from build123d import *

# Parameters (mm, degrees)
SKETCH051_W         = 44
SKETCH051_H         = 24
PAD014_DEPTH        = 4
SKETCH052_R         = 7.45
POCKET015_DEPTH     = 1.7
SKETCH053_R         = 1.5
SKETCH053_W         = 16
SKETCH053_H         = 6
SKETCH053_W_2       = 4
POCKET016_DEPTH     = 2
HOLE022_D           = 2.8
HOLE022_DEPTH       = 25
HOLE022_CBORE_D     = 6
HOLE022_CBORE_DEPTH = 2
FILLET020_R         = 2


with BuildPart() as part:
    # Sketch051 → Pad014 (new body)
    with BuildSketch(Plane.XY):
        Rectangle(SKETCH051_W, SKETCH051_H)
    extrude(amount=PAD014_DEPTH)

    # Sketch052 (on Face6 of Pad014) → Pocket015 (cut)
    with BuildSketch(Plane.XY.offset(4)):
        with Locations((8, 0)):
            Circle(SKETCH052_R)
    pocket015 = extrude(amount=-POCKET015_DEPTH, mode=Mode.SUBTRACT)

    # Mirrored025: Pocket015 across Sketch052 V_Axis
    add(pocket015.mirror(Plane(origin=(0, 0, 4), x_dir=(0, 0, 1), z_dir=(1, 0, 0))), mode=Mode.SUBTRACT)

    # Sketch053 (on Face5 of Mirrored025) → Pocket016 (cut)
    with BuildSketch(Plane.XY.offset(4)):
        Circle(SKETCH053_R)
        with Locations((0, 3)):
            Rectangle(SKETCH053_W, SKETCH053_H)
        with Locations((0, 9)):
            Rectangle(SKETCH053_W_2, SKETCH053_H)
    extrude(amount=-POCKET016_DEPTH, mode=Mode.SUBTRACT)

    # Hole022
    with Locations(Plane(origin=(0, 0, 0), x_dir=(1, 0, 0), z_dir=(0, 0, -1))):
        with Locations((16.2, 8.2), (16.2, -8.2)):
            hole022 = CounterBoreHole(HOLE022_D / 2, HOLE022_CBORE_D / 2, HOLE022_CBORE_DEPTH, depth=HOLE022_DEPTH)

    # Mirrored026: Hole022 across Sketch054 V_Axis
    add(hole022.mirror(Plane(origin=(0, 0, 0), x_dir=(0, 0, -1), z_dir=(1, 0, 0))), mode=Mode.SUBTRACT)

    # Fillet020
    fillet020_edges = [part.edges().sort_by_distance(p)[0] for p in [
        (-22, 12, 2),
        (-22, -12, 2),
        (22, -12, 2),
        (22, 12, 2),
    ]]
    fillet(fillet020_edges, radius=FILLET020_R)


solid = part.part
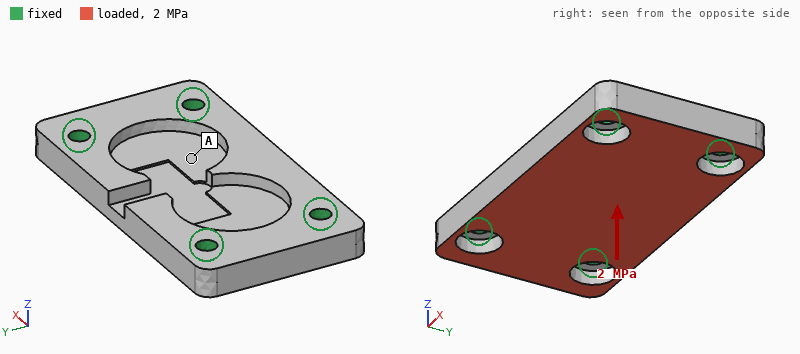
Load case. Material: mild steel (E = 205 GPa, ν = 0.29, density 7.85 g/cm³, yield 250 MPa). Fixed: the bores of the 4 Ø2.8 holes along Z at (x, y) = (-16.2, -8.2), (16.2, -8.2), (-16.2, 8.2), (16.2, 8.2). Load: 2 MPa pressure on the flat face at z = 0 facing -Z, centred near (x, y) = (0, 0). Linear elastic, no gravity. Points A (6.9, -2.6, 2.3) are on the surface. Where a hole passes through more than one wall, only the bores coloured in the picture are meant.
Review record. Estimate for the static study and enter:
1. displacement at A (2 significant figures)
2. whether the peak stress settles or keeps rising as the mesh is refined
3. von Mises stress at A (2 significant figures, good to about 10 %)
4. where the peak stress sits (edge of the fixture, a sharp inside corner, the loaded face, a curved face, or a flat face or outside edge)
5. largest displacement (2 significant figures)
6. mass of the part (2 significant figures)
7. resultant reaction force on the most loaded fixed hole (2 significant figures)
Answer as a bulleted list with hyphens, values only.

- 11 µm
- keeps rising
- 21 MPa
- edge of the fixture
- 16 µm
- 25 g
- 750 N
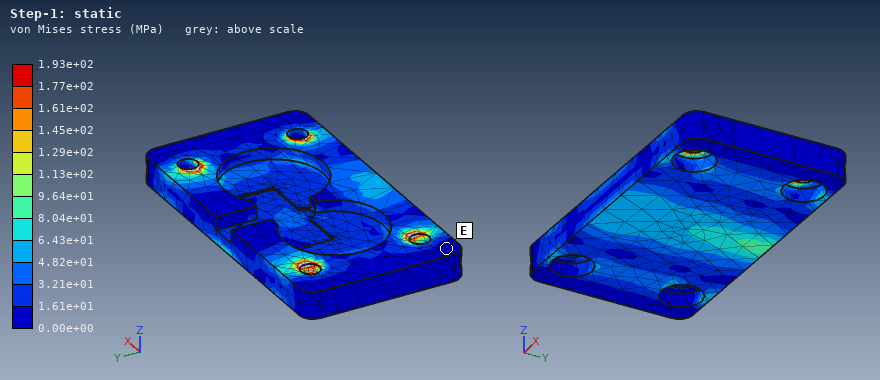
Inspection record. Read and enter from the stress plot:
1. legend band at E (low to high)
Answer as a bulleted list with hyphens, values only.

- 0.00e+00 to 1.61e+01 MPa
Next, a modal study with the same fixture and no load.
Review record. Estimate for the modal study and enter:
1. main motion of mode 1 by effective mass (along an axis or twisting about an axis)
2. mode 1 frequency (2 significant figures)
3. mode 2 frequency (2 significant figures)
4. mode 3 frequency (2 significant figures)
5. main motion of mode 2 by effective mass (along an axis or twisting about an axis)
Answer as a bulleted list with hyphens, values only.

- along Z
- 14 kHz
- 18 kHz
- 30 kHz
- twisting about X
